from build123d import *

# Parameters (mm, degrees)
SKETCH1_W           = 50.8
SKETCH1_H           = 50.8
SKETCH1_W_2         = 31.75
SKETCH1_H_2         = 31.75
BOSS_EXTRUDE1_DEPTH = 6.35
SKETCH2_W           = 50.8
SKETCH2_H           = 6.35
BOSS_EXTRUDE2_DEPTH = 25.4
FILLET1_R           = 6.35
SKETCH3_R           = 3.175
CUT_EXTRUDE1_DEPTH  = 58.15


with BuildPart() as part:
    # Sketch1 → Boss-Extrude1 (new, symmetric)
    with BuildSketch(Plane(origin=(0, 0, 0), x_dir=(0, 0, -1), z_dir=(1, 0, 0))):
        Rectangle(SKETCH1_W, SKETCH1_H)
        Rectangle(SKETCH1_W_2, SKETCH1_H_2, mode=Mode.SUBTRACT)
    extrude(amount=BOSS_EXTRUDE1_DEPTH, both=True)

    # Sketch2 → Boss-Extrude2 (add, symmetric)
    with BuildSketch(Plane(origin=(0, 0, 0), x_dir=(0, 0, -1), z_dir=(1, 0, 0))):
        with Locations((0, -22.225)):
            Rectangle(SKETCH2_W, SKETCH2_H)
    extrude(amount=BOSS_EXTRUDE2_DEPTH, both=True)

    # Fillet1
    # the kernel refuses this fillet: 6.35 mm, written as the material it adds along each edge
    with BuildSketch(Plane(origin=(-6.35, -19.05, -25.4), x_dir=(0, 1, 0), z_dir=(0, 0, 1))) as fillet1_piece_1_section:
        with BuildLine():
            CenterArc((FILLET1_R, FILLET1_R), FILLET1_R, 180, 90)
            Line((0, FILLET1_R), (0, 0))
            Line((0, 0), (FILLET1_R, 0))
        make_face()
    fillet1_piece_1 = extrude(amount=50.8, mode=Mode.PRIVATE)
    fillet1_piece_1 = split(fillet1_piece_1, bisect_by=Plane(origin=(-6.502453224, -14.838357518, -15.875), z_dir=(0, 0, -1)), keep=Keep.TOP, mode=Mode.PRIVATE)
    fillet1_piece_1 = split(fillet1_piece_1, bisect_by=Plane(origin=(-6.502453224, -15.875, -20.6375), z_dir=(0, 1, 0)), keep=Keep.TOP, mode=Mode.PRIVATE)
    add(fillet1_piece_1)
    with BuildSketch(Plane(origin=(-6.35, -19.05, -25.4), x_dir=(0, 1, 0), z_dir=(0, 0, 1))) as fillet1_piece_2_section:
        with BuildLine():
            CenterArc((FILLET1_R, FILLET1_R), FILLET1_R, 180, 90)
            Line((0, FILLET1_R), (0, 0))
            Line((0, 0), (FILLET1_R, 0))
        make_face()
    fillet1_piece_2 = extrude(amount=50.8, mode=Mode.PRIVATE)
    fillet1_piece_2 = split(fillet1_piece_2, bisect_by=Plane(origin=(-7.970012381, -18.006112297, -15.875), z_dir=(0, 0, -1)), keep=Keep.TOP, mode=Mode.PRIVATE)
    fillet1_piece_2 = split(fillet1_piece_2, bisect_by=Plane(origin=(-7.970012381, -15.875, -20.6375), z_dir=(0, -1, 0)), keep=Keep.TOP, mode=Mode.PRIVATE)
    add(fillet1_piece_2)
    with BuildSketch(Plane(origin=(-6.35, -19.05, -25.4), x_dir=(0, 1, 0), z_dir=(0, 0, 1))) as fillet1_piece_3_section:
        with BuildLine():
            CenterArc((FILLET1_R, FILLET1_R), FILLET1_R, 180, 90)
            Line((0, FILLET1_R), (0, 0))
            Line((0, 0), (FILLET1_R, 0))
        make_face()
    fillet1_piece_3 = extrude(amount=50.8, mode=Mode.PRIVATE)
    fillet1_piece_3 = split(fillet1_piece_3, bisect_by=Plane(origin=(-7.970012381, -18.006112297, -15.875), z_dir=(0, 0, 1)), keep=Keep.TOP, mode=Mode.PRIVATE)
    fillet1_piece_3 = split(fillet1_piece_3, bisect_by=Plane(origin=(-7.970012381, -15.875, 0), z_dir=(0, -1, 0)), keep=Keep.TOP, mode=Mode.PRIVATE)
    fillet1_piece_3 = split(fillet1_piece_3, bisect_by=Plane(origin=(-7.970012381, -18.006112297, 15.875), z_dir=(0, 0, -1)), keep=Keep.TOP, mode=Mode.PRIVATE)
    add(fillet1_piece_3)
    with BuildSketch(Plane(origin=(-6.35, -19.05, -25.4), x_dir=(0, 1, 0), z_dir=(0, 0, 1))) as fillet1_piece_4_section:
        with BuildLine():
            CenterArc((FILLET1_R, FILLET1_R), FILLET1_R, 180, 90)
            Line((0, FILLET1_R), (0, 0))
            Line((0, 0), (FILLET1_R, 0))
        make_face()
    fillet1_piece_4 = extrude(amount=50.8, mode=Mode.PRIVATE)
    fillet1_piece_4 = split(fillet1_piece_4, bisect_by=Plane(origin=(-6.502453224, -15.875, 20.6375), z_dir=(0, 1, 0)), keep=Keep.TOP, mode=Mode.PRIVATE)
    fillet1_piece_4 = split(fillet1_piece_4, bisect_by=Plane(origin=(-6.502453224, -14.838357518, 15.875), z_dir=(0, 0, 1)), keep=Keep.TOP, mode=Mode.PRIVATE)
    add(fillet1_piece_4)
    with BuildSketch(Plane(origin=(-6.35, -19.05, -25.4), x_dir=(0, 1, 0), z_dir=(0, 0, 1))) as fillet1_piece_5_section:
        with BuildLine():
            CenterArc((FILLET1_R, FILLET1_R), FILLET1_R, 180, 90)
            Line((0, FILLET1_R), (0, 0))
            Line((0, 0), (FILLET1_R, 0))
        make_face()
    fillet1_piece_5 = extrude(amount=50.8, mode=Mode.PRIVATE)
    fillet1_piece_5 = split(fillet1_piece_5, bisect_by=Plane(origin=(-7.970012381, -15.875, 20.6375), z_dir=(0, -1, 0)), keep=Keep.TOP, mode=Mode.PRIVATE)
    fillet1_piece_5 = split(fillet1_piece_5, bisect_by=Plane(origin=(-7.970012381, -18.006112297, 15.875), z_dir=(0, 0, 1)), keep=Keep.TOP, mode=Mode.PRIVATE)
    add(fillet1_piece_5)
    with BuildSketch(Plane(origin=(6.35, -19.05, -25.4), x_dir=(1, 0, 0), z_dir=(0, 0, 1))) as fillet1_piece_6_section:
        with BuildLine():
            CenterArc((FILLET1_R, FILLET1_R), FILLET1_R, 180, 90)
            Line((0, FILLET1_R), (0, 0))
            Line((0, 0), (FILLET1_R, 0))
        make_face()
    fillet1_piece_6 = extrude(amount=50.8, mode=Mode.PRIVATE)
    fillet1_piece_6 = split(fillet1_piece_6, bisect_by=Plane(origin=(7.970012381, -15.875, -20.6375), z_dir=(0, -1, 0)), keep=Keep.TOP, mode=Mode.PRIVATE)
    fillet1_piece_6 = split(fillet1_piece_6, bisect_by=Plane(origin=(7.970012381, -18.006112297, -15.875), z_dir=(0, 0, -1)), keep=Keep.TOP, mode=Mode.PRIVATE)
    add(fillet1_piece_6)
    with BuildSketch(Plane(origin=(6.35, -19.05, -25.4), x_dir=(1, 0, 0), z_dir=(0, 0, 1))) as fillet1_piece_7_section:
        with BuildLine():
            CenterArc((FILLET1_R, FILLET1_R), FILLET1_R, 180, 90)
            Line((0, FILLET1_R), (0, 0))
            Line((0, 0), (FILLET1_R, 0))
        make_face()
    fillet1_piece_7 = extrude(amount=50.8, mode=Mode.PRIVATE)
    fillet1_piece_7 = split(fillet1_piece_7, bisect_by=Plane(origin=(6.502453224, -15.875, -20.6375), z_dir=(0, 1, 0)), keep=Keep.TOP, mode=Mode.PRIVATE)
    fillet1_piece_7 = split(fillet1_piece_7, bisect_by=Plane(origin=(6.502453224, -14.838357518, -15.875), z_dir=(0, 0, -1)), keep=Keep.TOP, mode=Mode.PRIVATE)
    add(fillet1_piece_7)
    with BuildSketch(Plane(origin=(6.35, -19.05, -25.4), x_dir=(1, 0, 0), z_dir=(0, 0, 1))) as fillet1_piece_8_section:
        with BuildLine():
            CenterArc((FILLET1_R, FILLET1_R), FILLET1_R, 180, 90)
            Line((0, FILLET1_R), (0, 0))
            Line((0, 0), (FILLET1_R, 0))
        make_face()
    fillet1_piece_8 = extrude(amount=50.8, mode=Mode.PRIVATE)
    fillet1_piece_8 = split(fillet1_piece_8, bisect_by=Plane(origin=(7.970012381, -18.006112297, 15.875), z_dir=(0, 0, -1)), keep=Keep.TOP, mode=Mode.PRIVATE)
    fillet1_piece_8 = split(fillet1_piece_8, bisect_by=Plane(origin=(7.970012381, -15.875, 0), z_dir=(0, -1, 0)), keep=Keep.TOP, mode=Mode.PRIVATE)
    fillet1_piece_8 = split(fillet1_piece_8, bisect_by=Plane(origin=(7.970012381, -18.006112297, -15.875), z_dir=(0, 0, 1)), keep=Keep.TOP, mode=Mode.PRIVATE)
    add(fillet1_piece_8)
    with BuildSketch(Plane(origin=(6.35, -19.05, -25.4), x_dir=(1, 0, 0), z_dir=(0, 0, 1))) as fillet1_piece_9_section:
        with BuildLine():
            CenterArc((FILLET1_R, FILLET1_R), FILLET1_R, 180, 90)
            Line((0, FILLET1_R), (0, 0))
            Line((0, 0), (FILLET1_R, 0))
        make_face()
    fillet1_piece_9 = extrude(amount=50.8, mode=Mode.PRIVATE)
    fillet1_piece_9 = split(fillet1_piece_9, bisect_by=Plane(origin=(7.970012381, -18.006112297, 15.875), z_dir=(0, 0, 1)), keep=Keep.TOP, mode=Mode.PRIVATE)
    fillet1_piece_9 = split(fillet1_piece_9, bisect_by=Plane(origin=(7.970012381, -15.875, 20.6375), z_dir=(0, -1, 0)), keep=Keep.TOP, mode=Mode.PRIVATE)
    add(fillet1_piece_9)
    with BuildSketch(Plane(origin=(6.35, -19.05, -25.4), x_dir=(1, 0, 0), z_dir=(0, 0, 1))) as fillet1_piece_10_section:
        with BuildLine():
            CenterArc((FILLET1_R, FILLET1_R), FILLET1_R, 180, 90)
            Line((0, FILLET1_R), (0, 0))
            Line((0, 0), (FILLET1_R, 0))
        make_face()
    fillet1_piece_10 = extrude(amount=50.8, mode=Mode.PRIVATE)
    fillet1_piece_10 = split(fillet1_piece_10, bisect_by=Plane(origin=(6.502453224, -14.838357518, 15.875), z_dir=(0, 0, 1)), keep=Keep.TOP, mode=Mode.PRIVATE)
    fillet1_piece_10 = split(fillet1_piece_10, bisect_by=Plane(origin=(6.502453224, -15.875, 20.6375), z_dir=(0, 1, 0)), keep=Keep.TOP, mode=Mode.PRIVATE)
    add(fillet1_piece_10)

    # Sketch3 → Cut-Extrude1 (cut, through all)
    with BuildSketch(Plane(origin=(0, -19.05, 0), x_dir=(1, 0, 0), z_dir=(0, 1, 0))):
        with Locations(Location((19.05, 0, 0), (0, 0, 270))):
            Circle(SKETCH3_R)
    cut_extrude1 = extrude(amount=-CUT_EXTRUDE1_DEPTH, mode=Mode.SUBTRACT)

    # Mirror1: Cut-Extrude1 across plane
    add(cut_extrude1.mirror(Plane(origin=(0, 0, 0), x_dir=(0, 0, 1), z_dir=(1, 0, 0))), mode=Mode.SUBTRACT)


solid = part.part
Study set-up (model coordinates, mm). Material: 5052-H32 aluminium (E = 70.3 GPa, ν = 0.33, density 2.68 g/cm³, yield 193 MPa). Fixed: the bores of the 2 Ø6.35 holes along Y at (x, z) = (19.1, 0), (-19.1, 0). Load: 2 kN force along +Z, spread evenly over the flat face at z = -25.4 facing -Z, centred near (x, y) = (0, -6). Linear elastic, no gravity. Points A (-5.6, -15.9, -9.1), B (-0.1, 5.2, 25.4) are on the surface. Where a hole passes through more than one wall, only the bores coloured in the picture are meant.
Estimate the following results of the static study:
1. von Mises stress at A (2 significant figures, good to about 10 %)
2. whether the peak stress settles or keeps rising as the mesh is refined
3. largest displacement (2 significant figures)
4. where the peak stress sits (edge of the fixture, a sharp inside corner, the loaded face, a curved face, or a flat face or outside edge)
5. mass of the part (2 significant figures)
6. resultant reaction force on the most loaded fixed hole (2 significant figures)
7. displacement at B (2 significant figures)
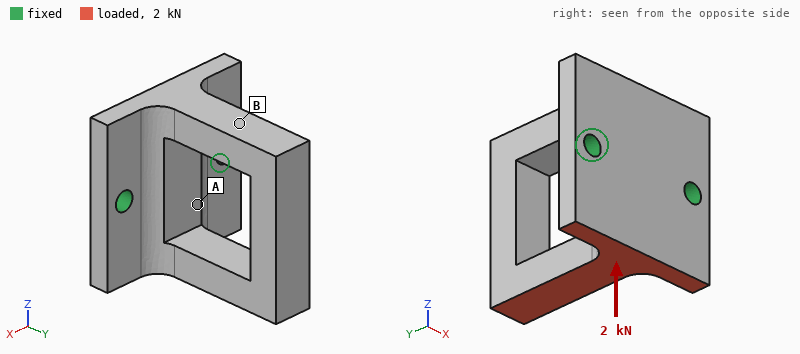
34 MPa
keeps rising
0.18 mm
edge of the fixture
88 g
1.0 kN
0.12 mm
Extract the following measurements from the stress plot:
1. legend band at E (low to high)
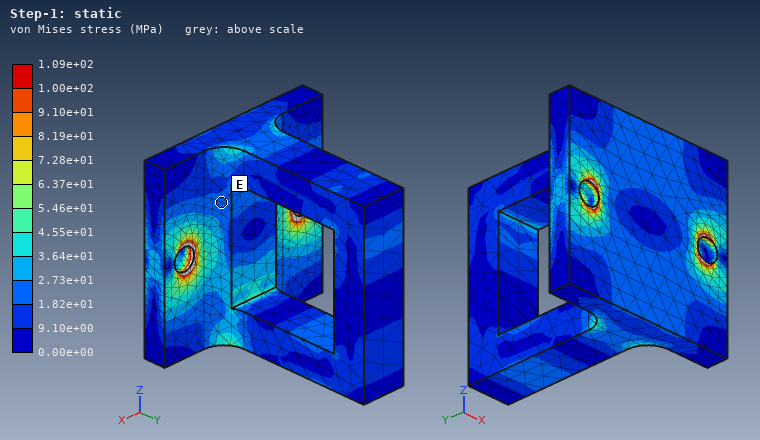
1.82e+01 to 2.73e+01 MPa
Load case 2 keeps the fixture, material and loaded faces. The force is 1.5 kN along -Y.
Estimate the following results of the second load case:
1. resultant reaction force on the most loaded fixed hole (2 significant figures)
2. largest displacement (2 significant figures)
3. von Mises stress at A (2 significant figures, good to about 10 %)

830 N
0.16 mm
35 MPa
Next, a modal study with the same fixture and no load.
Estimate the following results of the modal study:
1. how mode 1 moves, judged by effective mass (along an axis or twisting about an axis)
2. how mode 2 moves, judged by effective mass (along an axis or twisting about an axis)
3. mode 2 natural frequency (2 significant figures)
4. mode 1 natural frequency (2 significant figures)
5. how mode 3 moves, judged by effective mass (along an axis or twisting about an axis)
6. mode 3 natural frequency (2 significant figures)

along Z
along X
2800 Hz
2100 Hz
twisting about Y
5400 Hz
